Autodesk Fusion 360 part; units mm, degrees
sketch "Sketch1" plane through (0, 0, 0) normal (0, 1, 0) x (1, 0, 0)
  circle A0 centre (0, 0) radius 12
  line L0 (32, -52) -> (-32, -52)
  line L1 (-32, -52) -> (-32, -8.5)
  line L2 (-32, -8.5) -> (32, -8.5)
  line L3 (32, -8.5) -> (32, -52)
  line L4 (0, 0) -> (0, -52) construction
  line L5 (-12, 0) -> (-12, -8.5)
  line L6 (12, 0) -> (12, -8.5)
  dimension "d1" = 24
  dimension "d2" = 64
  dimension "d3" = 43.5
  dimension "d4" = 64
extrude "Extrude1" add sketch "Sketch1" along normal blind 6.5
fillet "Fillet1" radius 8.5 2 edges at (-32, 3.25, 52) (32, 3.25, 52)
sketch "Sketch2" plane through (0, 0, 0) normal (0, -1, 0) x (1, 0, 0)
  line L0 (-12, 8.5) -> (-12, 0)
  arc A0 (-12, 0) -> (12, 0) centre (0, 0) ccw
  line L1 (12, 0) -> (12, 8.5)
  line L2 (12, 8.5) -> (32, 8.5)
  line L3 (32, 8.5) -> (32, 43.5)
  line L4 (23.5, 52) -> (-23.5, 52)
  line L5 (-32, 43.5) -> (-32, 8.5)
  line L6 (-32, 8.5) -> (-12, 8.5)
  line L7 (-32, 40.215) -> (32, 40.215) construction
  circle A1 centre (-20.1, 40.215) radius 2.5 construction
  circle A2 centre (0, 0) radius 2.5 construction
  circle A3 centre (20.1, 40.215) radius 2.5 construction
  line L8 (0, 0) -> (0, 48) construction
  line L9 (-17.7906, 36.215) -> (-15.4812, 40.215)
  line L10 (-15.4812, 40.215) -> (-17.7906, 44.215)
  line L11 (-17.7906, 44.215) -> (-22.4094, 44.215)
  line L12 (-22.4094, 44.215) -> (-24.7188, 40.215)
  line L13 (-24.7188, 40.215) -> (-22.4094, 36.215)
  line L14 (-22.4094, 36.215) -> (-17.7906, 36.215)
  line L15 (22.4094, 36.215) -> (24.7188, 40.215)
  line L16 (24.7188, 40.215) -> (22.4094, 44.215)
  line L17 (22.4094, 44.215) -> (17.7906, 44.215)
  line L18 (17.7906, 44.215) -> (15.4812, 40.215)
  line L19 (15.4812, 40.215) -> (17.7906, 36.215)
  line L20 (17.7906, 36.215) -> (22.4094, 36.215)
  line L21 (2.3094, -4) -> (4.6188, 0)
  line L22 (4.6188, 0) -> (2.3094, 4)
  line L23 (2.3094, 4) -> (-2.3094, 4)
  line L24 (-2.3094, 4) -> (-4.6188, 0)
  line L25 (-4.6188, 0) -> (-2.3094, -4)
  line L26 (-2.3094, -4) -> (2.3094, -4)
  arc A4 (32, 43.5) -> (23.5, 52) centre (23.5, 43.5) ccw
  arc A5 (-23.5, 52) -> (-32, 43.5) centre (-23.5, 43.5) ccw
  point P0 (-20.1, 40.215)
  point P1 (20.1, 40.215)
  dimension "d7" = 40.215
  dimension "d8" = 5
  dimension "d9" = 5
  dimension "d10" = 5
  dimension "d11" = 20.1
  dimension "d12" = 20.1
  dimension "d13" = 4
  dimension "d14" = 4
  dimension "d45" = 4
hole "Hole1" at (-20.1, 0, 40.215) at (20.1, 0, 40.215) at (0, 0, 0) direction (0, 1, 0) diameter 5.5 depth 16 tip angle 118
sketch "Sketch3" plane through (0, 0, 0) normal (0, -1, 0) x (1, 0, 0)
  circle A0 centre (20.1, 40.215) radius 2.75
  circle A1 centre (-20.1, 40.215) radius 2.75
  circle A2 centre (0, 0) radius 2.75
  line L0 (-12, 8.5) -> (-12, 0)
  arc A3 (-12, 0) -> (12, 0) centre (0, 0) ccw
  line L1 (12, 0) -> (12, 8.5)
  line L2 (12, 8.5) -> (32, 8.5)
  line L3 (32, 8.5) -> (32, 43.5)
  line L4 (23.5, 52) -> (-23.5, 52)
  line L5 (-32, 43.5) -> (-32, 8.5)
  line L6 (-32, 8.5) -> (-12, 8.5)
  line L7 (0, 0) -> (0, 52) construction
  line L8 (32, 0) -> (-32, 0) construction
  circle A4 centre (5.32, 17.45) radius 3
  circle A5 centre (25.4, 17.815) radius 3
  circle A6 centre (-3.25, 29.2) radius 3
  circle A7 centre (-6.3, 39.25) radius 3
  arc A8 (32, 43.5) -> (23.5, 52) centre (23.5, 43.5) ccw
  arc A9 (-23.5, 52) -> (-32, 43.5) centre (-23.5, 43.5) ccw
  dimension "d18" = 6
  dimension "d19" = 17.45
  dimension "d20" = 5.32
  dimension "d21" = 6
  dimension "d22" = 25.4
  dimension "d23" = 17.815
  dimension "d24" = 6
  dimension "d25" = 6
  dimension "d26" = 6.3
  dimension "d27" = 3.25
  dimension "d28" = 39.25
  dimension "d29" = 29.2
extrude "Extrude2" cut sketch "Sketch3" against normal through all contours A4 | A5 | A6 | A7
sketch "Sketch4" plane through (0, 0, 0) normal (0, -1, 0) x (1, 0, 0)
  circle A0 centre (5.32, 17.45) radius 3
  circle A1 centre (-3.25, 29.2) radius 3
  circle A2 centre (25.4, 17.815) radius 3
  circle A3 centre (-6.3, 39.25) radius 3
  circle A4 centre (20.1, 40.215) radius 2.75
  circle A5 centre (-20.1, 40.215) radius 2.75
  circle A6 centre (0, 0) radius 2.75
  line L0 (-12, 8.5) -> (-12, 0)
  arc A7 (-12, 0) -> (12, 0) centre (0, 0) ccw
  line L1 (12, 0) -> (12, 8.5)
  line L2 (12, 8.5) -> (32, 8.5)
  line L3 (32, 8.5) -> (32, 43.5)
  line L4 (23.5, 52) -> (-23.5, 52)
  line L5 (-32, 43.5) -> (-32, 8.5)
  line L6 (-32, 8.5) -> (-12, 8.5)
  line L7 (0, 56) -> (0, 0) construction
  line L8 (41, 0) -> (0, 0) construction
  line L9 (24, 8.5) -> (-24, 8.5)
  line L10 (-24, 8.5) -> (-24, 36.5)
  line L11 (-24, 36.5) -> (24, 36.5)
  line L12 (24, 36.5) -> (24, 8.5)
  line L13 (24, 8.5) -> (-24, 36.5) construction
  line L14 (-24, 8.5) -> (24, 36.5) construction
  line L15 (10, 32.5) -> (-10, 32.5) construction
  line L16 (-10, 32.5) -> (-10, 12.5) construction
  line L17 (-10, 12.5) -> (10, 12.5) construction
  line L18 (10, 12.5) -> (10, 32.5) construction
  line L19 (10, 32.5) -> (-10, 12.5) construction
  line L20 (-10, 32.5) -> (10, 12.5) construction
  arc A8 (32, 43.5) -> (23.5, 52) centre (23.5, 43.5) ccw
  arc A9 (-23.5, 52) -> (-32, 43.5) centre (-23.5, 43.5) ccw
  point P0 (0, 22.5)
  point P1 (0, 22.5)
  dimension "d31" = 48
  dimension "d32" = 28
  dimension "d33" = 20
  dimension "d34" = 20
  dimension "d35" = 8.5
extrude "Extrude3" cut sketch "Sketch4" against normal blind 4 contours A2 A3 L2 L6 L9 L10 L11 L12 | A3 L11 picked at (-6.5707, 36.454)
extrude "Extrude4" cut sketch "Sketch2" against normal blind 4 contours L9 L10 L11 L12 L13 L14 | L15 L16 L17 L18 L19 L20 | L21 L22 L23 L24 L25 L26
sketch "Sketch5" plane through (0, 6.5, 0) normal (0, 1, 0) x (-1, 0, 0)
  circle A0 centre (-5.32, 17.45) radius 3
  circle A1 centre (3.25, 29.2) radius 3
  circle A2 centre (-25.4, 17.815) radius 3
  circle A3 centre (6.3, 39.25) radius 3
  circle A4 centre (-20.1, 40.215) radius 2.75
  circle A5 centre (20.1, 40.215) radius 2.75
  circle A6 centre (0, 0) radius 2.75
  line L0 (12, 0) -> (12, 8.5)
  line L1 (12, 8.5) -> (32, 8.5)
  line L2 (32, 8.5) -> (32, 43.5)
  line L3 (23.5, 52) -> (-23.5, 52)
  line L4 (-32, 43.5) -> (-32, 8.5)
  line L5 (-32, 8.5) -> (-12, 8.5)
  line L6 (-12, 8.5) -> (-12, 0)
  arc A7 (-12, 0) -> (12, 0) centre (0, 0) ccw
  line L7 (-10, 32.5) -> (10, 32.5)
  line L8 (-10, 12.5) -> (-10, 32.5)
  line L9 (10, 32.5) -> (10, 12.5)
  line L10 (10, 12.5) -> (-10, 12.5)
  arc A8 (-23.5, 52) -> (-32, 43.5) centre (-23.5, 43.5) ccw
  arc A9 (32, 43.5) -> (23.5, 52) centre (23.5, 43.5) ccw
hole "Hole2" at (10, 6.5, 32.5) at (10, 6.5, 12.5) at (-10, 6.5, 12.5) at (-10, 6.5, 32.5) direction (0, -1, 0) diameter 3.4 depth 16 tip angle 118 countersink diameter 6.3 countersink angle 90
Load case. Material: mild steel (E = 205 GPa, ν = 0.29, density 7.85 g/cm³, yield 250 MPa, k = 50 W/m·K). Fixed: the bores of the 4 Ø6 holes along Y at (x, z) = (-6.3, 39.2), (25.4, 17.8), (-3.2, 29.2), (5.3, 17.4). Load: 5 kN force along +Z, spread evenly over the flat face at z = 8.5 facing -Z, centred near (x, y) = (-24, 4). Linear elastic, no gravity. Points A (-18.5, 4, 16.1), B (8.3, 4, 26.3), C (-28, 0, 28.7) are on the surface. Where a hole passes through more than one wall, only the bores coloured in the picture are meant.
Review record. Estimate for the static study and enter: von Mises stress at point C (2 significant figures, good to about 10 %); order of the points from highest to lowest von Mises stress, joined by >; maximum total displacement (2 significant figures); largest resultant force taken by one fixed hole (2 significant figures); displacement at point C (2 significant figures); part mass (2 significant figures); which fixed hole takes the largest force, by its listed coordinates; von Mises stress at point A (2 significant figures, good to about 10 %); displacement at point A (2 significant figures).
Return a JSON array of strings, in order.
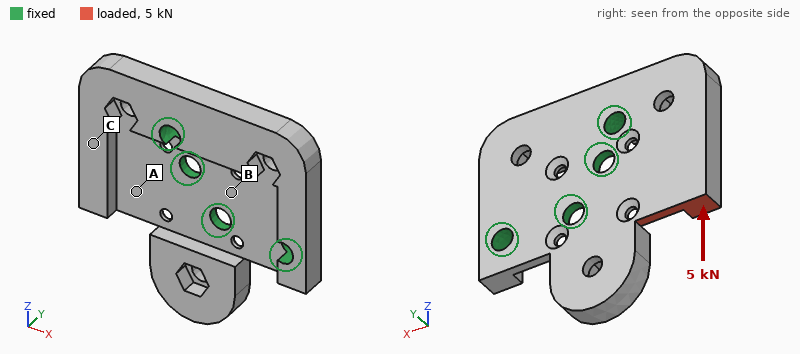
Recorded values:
["63 MPa", "A > C > B", "41 µm", "4.2 kN", "24 µm", "110 g", "(-6.3, 39.2)", "96 MPa", "21 µm"]
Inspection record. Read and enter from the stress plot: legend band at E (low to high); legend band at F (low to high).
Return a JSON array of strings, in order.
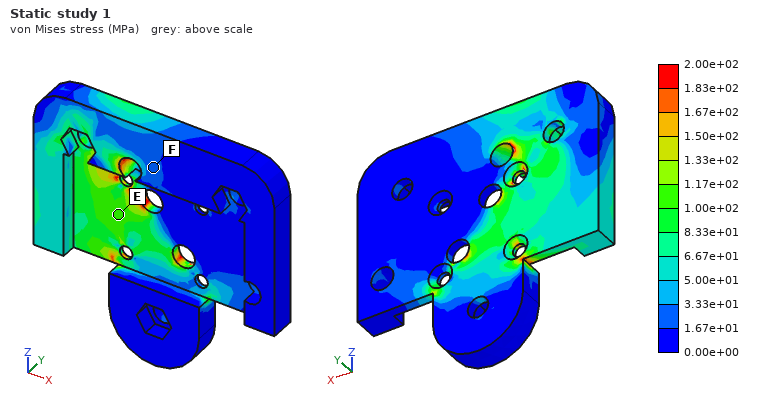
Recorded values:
["1.00e+02 to 1.17e+02 MPa", "1.67e+01 to 3.33e+01 MPa"]
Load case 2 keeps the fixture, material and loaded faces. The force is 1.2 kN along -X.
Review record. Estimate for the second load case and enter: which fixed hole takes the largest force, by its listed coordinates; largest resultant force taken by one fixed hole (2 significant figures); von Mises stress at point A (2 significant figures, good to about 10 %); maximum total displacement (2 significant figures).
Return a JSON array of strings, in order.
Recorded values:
["(5.3, 17.4)", "890 N", "54 MPa", "32 µm"]
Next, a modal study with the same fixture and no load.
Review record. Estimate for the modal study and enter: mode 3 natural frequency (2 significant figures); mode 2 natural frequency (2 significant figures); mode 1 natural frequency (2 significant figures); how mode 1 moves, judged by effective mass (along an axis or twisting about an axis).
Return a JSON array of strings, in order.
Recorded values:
["7000 Hz", "3500 Hz", "2100 Hz", "along Y"]
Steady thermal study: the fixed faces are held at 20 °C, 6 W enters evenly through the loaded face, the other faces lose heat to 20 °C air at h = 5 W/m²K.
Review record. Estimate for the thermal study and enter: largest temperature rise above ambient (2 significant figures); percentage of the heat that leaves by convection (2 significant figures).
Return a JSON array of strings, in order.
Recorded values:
["39 K", "4.0 %"]
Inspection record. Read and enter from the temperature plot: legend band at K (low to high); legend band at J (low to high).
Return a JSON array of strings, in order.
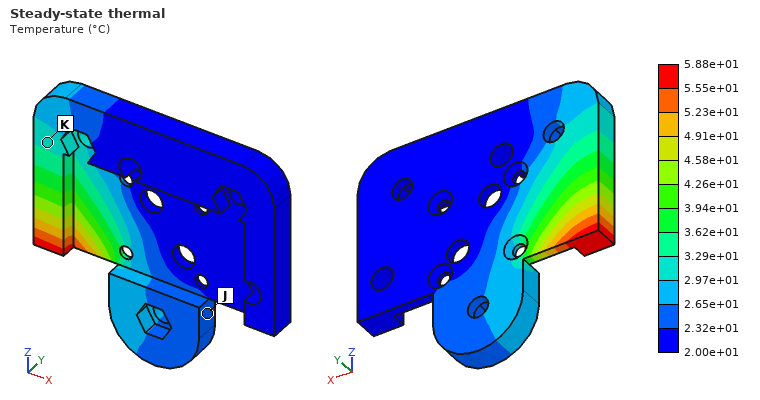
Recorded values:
["2.97e+01 to 3.29e+01 °C", "2.32e+01 to 2.65e+01 °C"]
